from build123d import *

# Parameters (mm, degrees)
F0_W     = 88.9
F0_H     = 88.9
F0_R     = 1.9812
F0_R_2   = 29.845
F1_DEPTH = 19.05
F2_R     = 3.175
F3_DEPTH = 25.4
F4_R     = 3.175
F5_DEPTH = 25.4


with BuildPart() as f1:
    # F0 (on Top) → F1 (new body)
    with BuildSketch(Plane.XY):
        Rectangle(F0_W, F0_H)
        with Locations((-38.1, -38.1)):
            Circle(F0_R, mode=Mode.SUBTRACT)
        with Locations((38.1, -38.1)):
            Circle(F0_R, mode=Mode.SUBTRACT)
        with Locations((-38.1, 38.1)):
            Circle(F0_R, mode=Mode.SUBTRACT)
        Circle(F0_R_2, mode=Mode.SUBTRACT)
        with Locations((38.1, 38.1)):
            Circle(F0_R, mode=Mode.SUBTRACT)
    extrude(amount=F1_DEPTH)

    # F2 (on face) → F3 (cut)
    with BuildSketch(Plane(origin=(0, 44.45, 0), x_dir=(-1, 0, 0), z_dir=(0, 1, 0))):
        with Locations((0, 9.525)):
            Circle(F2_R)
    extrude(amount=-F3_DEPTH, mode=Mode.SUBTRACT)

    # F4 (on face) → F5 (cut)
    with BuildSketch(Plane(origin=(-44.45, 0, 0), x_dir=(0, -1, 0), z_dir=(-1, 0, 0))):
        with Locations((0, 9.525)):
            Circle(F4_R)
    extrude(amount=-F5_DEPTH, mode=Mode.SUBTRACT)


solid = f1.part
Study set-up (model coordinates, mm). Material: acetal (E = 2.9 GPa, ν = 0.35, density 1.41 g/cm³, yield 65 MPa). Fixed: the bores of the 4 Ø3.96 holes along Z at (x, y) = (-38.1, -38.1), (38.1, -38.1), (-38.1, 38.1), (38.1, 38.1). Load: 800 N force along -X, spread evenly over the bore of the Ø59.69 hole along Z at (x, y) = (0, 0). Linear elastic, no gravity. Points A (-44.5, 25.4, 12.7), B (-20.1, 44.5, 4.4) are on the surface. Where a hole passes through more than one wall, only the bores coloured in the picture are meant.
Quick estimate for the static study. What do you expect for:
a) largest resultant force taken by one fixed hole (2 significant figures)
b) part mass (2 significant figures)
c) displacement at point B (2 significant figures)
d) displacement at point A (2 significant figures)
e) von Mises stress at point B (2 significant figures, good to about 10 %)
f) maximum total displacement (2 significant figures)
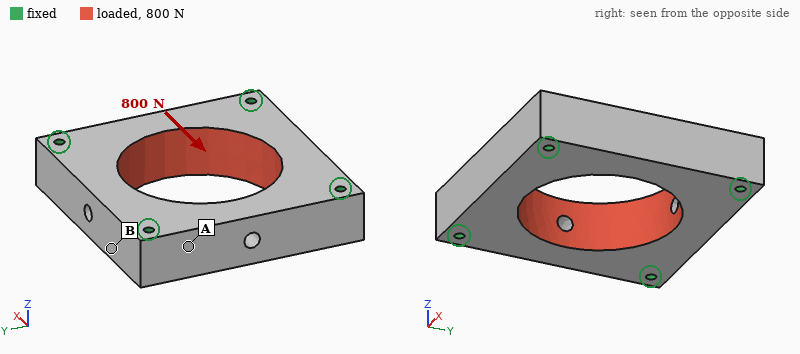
210 N
130 g
5.0 µm
8.9 µm
0.87 MPa
21 µm
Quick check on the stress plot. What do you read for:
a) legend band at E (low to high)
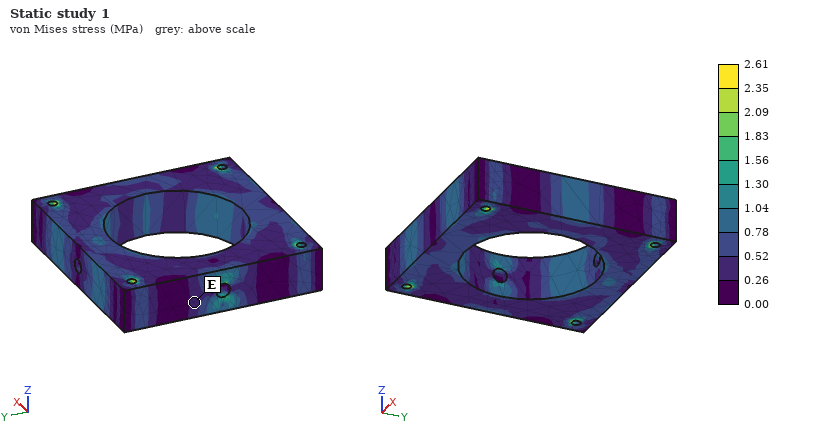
0.26 to 0.52 MPa
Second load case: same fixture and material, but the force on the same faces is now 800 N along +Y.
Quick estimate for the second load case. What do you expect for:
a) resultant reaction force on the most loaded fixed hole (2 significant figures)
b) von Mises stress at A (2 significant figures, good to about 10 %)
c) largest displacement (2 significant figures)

210 N
0.81 MPa
21 µm
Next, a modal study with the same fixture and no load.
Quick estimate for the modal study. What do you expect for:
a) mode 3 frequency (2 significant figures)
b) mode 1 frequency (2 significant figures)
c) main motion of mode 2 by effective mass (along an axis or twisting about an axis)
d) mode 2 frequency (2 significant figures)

3500 Hz
2100 Hz
along Z
3000 Hz
